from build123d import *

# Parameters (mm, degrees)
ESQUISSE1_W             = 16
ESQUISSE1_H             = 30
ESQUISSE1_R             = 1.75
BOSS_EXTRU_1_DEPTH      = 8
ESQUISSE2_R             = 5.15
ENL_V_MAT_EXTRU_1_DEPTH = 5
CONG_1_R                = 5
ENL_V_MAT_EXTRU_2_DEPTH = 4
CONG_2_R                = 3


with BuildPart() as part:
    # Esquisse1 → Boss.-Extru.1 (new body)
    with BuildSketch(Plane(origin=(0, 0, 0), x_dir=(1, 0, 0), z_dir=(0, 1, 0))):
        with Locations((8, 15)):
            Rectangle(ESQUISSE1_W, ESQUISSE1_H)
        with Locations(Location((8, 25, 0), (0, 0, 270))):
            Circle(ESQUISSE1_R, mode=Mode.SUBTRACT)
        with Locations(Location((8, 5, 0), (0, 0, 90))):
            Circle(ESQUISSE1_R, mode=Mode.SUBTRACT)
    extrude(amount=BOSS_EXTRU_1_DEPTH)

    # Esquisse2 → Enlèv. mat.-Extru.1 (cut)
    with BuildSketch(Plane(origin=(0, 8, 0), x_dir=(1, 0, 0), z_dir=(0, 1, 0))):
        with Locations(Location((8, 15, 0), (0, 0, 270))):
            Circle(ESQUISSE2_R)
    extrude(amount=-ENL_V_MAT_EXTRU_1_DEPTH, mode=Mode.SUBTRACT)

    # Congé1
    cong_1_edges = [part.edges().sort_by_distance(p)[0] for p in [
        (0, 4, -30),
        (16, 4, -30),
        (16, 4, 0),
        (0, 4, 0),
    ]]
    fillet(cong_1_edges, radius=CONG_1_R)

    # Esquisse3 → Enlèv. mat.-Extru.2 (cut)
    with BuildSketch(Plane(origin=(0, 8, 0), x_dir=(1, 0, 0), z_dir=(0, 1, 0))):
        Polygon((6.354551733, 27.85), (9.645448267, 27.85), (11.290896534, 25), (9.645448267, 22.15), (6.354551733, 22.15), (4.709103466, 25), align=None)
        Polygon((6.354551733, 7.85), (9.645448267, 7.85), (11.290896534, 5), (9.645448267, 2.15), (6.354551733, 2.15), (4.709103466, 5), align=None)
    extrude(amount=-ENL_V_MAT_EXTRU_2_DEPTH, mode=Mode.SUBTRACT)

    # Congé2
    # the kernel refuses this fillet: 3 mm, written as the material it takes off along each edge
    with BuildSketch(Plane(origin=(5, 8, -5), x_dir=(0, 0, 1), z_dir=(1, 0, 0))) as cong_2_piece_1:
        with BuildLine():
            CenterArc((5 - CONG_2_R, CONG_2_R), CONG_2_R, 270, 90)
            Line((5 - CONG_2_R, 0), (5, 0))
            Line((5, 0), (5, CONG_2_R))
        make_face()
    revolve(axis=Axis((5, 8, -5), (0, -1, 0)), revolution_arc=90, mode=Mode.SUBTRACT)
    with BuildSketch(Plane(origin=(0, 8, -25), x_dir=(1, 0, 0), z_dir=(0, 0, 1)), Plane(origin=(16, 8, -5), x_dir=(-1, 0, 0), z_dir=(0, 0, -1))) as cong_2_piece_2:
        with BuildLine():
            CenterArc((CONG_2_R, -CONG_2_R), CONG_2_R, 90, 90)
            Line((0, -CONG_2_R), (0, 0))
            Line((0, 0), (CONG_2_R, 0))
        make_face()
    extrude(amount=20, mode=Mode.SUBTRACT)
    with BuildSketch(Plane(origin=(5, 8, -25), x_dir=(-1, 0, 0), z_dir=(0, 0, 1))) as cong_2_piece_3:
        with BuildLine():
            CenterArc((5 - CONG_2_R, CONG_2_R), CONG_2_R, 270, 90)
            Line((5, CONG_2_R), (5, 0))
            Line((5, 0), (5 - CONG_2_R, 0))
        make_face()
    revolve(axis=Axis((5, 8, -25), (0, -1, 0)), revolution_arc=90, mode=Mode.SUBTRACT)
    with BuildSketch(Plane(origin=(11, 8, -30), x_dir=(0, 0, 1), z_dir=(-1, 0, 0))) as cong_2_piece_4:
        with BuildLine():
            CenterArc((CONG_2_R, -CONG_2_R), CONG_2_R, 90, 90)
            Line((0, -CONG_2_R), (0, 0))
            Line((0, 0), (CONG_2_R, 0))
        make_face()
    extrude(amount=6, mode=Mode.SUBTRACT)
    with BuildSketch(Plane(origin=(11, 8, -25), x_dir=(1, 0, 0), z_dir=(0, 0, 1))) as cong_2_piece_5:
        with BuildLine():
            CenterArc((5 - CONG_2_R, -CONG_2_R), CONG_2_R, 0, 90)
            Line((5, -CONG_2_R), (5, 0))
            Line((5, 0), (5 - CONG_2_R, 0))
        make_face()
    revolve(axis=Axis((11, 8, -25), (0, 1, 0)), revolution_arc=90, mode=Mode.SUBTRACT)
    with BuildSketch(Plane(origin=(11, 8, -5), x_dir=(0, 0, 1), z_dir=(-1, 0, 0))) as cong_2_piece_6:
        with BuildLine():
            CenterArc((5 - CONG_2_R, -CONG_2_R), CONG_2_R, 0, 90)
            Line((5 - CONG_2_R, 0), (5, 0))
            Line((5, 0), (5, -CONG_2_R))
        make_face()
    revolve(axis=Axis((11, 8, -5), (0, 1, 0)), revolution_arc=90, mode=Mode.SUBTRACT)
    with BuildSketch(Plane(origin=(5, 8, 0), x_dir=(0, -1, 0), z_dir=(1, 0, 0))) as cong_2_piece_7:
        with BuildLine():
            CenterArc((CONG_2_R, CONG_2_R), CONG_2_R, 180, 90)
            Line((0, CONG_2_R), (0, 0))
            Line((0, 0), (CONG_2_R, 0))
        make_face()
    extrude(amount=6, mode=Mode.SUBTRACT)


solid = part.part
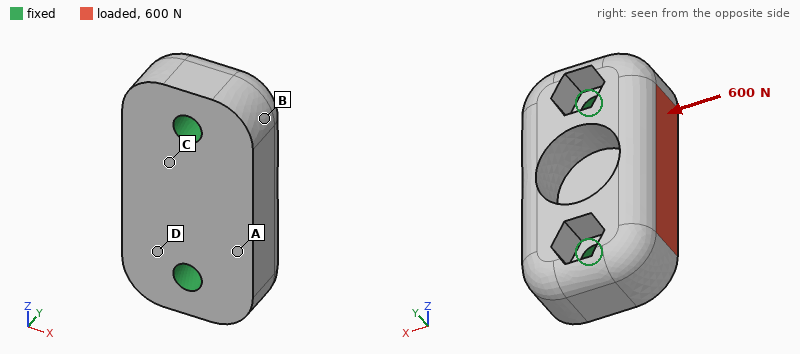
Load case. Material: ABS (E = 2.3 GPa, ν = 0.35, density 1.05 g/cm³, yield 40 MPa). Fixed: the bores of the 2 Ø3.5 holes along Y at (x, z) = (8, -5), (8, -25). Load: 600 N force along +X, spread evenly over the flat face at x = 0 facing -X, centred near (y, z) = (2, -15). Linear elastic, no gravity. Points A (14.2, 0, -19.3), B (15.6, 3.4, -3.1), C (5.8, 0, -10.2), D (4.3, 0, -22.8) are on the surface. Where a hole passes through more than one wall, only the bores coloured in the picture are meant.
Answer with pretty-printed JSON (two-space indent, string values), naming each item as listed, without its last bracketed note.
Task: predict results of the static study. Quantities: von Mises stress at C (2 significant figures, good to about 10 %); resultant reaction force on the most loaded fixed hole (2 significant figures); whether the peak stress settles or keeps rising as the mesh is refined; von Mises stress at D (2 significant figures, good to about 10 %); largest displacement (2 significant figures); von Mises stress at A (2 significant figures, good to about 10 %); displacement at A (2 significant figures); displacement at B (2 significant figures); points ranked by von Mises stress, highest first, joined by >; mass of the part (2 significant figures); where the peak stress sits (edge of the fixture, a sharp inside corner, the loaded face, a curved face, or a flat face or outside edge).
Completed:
{
  "von Mises stress at C": "6.0 MPa",
  "resultant reaction force on the most loaded fixed hole": "310 N",
  "whether the peak stress settles or keeps rising as the mesh is refined": "keeps rising",
  "von Mises stress at D": "8.6 MPa",
  "largest displacement": "52 µm",
  "von Mises stress at A": "3.4 MPa",
  "displacement at A": "20 µm",
  "displacement at B": "14 µm",
  "points ranked by von Mises stress, highest first, joined by >": "D > C > A > B",
  "mass of the part": "2.9 g",
  "where the peak stress sits": "edge of the fixture"
}
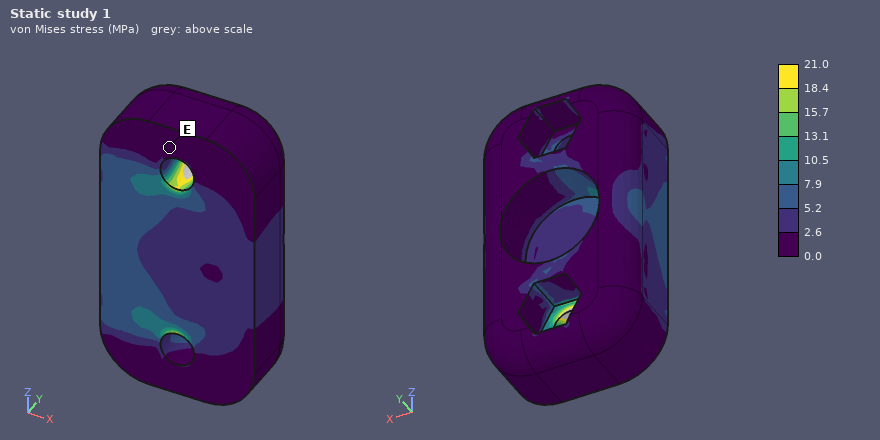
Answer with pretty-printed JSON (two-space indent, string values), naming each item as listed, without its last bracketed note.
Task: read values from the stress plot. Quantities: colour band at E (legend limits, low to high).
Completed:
{
  "colour band at E": "0.0 to 2.6 MPa"
}
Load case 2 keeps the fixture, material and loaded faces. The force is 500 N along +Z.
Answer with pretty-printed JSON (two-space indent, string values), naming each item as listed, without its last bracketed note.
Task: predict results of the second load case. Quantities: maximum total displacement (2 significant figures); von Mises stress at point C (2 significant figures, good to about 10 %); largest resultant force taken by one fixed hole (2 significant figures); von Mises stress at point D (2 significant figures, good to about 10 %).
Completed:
{
  "maximum total displacement": "47 µm",
  "von Mises stress at point C": "8.0 MPa",
  "largest resultant force taken by one fixed hole": "300 N",
  "von Mises stress at point D": "8.5 MPa"
}
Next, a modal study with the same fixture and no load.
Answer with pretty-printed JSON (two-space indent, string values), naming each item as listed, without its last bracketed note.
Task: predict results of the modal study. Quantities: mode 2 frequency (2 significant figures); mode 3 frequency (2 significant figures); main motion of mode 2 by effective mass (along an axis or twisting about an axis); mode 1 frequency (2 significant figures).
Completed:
{
  "mode 2 frequency": "11 kHz",
  "mode 3 frequency": "13 kHz",
  "main motion of mode 2 by effective mass": "along Y",
  "mode 1 frequency": "8100 Hz"
}
